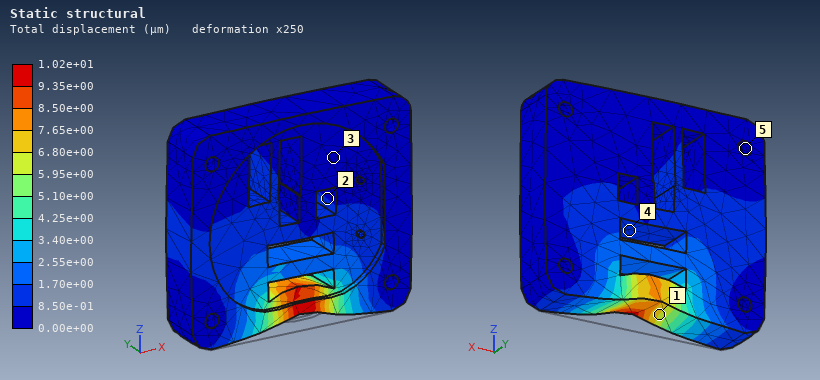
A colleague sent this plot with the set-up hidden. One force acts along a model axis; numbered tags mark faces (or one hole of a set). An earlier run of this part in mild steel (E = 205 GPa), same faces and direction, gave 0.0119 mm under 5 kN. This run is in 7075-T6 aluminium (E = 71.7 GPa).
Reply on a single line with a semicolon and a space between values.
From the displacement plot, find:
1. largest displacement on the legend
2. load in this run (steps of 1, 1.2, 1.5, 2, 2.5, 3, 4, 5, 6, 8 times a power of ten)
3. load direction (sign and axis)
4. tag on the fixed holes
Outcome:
1.02e+01 µm; 1.5 kN; +Z; 5
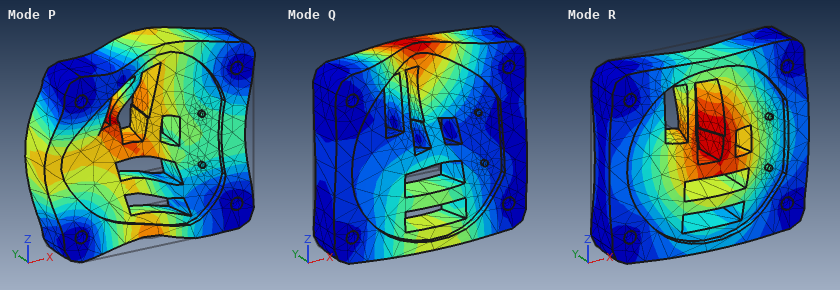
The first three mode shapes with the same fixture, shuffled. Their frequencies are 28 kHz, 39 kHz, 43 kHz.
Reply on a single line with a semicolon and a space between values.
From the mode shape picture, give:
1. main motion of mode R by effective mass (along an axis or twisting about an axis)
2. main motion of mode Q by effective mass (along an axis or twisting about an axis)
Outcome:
along Y; twisting about X
